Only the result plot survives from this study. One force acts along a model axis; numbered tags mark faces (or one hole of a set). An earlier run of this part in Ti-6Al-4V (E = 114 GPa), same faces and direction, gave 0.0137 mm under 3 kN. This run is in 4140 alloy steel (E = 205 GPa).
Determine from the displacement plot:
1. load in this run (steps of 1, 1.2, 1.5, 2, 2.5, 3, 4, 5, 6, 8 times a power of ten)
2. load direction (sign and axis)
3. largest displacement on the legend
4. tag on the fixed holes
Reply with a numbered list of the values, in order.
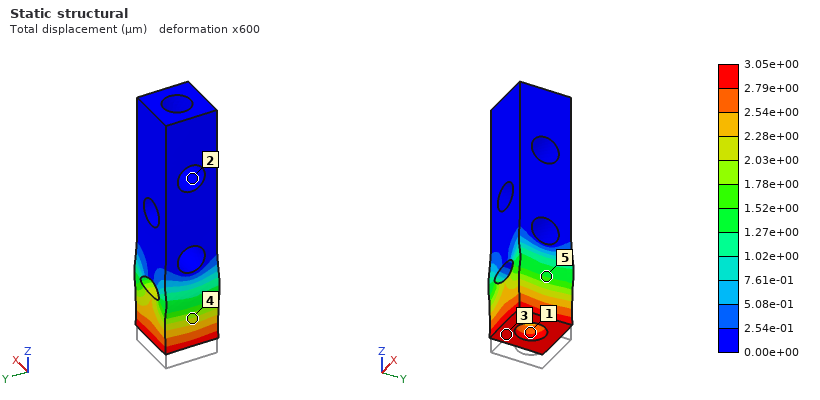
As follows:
1. 1.2 kN
2. +Z
3. 3.05e+00 µm
4. 2
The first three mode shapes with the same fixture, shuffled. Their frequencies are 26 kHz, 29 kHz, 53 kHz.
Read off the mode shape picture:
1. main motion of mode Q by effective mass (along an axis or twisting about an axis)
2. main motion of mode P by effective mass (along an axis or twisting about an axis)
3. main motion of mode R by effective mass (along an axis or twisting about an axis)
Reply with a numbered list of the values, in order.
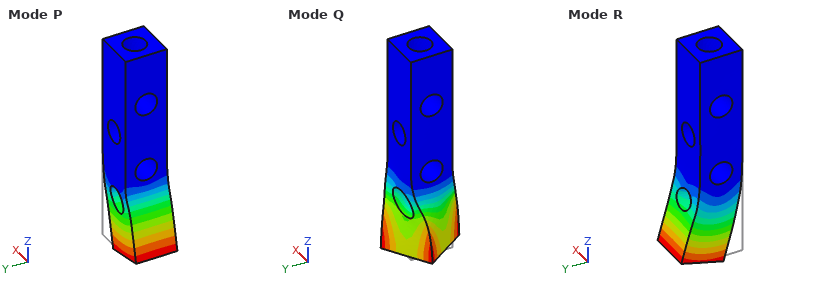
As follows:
1. twisting about Z
2. along X
3. along Y
